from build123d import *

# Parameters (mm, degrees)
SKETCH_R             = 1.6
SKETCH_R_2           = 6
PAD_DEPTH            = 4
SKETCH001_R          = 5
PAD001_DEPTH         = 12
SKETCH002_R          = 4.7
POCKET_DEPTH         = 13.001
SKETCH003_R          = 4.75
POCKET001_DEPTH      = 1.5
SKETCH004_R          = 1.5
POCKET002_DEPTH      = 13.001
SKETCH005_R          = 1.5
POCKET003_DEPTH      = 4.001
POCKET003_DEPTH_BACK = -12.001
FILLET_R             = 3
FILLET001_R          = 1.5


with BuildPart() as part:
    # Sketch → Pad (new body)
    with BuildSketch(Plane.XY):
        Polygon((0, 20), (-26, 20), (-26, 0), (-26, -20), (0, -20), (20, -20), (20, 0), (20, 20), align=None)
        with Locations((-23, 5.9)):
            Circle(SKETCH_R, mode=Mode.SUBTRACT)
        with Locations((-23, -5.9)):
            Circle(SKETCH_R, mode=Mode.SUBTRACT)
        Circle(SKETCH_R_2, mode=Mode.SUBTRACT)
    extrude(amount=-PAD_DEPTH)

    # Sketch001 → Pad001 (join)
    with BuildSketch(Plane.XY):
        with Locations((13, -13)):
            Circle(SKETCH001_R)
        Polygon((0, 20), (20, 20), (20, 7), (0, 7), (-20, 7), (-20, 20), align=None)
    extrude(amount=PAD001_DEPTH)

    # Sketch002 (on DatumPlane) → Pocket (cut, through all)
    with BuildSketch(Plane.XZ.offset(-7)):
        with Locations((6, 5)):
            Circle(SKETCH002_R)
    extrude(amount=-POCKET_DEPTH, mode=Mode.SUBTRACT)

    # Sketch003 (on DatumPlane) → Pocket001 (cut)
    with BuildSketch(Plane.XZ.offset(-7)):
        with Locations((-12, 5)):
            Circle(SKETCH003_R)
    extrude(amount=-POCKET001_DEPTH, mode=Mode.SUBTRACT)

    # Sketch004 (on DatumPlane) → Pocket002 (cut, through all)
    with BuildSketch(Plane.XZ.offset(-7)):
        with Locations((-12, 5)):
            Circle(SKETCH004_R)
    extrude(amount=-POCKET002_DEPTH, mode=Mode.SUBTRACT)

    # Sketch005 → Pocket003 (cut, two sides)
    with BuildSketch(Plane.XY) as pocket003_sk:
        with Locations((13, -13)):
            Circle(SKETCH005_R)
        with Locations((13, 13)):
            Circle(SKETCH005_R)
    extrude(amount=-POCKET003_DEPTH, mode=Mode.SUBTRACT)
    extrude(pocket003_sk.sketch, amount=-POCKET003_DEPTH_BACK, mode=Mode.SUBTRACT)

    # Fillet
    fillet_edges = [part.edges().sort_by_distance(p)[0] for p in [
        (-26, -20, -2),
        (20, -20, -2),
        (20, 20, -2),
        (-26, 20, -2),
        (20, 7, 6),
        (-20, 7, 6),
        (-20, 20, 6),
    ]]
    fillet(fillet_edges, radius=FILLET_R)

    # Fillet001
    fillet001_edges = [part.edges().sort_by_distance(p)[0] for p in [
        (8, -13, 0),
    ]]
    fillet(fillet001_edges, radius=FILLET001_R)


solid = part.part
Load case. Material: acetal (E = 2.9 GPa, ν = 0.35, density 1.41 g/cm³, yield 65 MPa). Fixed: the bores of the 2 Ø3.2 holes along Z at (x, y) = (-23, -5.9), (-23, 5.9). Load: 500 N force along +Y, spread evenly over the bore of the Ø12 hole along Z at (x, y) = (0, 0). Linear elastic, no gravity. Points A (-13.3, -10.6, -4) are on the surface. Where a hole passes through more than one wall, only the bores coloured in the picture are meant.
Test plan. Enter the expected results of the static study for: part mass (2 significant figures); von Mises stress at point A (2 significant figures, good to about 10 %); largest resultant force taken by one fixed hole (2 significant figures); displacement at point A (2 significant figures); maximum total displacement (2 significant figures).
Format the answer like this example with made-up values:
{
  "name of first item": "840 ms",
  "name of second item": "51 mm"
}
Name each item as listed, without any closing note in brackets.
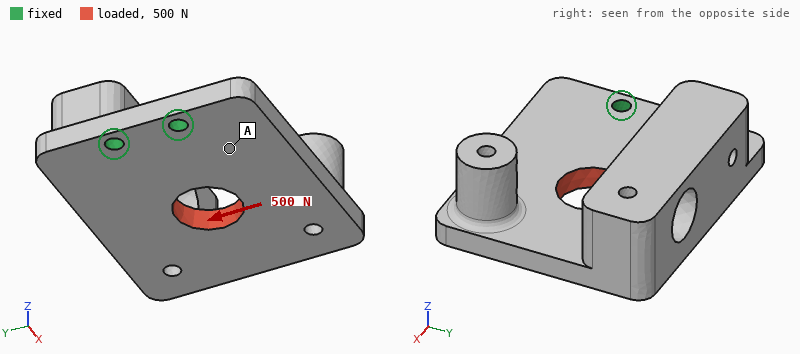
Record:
{
  "part mass": "18 g",
  "von Mises stress at point A": "6.7 MPa",
  "largest resultant force taken by one fixed hole": "800 N",
  "displacement at point A": "0.17 mm",
  "maximum total displacement": "0.66 mm"
}
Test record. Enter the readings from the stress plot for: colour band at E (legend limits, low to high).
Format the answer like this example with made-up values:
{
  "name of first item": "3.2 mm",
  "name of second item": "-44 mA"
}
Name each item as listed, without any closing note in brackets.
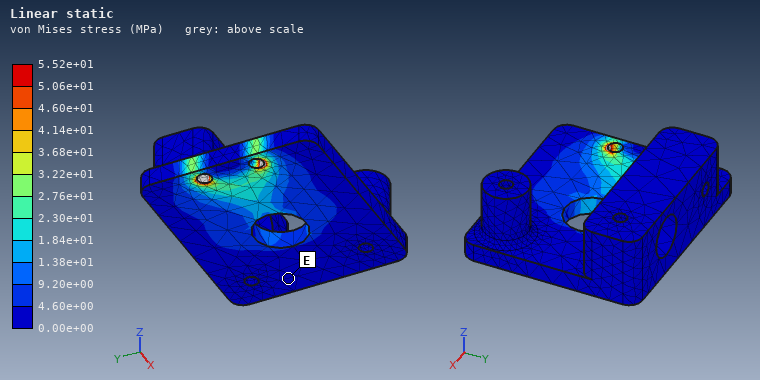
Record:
{
  "colour band at E": "0.00e+00 to 4.60e+00 MPa"
}
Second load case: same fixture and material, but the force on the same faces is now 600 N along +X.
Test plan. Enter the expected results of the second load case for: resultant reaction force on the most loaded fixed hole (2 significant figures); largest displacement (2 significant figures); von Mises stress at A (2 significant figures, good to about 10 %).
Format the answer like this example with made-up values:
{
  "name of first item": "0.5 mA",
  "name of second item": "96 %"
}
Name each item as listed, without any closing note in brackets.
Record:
{
  "resultant reaction force on the most loaded fixed hole": "300 N",
  "largest displacement": "87 µm",
  "von Mises stress at A": "5.2 MPa"
}
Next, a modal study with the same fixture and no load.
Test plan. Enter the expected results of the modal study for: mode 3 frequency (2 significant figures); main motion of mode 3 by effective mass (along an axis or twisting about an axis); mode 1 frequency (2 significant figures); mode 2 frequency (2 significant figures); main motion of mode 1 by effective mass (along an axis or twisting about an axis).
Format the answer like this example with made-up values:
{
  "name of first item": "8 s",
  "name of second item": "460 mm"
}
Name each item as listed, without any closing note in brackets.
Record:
{
  "mode 3 frequency": "1200 Hz",
  "main motion of mode 3 by effective mass": "along Y",
  "mode 1 frequency": "370 Hz",
  "mode 2 frequency": "760 Hz",
  "main motion of mode 1 by effective mass": "along Z"
}
